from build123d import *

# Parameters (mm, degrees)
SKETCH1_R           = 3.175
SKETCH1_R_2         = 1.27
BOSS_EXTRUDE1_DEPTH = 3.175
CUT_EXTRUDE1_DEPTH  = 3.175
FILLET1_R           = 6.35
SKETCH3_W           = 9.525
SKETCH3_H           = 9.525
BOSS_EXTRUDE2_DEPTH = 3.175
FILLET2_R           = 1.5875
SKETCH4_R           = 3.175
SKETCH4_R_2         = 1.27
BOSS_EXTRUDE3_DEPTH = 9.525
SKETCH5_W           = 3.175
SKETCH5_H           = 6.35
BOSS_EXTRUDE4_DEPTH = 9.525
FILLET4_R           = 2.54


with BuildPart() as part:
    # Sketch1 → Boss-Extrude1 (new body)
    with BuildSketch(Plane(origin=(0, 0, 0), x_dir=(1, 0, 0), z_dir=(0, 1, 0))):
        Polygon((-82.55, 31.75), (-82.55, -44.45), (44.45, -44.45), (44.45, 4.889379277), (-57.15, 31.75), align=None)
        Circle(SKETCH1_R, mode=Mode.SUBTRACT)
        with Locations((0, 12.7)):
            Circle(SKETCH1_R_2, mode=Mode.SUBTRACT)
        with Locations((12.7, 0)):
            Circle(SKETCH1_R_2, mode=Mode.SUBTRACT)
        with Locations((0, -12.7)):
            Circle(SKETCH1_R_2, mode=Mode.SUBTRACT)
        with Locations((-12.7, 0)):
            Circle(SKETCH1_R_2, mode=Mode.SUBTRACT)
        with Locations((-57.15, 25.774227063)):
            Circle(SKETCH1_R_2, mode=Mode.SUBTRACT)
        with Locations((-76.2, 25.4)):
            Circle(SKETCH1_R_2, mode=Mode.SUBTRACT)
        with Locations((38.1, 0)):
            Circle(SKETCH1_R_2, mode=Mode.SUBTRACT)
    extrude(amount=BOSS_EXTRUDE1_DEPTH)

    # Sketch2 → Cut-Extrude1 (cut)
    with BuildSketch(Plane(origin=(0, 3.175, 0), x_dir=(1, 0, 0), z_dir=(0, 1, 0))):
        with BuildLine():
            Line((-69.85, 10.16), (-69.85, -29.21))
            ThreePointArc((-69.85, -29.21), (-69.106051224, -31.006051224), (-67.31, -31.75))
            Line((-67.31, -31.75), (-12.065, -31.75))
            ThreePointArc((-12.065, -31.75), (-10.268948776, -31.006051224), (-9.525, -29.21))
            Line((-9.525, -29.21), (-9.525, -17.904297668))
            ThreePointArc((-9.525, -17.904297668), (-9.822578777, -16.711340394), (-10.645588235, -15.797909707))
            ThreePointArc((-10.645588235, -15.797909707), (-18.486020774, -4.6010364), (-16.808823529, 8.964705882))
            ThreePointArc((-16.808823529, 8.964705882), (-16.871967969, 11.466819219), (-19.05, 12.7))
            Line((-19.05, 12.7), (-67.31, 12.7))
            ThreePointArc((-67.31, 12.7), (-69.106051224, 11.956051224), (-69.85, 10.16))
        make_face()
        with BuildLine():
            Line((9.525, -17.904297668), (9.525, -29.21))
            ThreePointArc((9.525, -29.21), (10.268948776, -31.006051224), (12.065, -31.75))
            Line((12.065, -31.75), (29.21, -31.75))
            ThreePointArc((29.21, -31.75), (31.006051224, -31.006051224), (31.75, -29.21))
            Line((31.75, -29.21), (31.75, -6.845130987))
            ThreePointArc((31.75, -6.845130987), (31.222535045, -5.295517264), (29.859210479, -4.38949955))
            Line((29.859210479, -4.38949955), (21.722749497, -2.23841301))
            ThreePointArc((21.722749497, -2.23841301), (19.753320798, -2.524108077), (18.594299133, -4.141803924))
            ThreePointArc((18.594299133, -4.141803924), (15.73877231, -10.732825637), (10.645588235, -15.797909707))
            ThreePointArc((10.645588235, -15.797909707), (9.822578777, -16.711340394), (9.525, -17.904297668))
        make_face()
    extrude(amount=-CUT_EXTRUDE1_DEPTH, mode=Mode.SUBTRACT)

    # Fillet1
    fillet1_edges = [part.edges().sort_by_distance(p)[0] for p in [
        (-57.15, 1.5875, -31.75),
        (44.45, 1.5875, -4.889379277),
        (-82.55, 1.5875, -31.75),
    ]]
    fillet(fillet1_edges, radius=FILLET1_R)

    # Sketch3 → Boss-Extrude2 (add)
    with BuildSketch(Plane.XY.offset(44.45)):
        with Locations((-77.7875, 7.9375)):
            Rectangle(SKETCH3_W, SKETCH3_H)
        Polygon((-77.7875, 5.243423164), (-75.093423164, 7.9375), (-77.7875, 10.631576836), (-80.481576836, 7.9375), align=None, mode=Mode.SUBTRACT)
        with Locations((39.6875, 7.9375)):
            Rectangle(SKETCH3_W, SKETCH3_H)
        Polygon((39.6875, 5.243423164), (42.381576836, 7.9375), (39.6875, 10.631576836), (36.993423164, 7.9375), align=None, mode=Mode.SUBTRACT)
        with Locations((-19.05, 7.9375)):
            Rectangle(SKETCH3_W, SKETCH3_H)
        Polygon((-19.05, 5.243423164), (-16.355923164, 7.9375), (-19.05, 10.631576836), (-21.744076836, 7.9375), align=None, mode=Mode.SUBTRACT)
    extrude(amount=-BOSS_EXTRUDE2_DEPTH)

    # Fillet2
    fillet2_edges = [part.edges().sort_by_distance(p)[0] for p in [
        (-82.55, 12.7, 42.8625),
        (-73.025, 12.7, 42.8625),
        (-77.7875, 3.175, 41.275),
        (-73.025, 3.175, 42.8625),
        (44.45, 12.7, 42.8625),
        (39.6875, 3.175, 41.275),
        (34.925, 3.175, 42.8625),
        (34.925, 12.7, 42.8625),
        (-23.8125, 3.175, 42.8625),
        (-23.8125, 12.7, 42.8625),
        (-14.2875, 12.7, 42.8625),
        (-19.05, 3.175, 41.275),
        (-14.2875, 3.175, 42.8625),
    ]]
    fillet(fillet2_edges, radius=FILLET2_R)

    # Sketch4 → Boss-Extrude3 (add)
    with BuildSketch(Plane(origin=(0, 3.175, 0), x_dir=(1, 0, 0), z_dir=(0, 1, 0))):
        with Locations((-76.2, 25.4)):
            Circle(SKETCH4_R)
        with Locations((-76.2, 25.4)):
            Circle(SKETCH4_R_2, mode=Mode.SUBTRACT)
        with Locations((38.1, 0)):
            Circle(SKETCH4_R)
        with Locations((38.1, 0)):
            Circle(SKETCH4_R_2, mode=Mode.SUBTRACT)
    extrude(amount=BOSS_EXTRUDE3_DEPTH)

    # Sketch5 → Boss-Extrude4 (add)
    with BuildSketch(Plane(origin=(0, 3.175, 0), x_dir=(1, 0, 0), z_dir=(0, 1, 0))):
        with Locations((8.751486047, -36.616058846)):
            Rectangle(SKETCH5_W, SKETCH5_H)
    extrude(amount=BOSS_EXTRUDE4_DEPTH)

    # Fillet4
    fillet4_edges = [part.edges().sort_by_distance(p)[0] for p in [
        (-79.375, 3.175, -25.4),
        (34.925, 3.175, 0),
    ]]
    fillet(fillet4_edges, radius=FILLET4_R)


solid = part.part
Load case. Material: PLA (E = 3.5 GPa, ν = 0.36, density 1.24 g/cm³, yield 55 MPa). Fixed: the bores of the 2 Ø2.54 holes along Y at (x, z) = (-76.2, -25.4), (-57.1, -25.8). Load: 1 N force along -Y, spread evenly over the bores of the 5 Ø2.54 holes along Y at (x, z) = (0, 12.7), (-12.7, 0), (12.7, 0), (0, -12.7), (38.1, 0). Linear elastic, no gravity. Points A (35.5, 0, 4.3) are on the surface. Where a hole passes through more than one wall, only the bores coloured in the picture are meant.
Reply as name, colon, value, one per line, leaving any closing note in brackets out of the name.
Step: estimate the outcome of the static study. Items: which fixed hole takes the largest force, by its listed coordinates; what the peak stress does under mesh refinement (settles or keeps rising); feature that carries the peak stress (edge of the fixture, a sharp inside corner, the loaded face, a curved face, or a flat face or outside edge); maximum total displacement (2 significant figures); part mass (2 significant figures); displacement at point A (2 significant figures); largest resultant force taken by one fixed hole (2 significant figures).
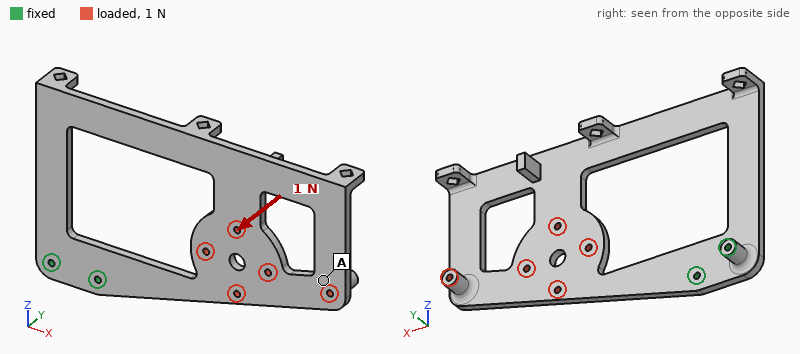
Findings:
which fixed hole takes the largest force, by its listed coordinates: (-57.1, -25.8)
what the peak stress does under mesh refinement: keeps rising
feature that carries the peak stress: edge of the fixture
maximum total displacement: 1.5 mm
part mass: 22 g
displacement at point A: 1.2 mm
largest resultant force taken by one fixed hole: 3.0 N
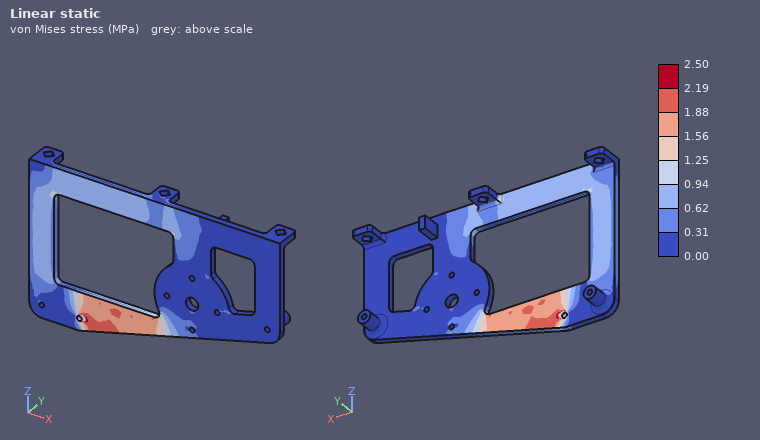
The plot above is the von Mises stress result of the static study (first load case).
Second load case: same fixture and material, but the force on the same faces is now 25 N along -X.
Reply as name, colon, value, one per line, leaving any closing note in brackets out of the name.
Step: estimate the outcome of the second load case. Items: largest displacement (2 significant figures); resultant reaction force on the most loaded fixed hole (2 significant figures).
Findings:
largest displacement: 1.6 mm
resultant reaction force on the most loaded fixed hole: 33 N
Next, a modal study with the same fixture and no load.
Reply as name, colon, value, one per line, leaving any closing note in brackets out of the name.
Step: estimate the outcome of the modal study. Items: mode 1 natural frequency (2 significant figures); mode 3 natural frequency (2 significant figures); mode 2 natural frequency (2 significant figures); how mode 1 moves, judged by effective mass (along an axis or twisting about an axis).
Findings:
mode 1 natural frequency: 43 Hz
mode 3 natural frequency: 260 Hz
mode 2 natural frequency: 120 Hz
how mode 1 moves, judged by effective mass: along Y
